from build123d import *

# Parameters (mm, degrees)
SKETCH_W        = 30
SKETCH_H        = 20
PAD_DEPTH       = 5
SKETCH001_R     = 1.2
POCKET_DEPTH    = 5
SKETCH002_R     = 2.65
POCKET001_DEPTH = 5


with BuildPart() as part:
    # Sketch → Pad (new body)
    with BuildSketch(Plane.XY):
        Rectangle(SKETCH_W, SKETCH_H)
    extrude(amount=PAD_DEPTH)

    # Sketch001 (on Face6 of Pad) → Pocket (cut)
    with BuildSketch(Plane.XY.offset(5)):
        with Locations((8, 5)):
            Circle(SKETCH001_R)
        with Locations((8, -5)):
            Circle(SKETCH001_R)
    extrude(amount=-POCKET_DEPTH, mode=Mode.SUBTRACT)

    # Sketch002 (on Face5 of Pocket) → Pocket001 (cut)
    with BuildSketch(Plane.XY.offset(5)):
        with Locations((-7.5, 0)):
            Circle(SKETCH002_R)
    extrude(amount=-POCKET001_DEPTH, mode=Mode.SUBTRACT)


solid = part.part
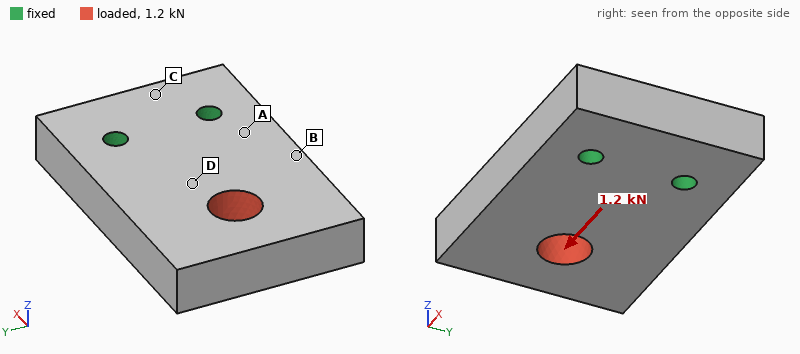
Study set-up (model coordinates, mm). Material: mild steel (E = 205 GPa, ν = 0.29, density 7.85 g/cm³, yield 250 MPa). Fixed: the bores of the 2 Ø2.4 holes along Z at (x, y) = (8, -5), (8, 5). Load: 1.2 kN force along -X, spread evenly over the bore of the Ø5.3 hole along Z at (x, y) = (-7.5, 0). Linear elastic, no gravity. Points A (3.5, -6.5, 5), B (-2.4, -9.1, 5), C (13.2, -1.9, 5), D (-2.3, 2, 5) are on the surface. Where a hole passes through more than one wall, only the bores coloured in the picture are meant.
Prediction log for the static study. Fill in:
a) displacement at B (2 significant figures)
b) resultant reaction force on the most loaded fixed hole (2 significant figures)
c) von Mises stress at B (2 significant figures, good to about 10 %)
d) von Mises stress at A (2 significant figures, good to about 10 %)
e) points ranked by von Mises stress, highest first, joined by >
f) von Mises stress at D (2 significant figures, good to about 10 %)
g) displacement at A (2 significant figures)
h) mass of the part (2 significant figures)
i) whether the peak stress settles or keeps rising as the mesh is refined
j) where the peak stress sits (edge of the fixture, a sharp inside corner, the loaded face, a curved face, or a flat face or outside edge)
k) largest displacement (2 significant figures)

0.69 µm
610 N
7.2 MPa
13 MPa
D > A > B > C
17 MPa
0.36 µm
22 g
keeps rising
edge of the fixture
1.7 µm
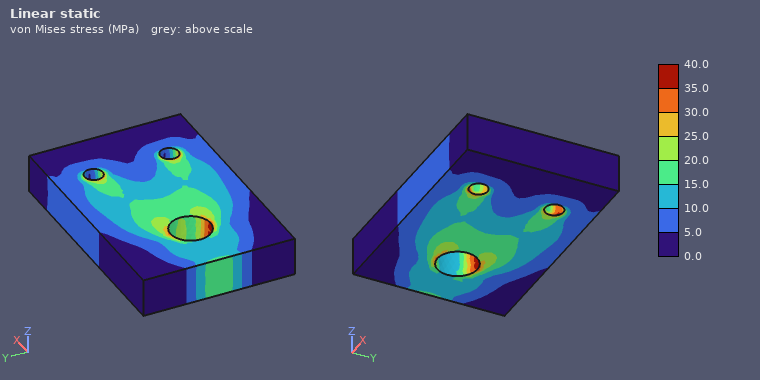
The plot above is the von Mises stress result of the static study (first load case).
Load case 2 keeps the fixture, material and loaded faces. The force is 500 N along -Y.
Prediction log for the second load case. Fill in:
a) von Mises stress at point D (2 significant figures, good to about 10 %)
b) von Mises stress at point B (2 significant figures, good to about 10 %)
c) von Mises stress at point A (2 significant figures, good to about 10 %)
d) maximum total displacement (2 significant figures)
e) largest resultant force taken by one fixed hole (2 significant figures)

14 MPa
7.8 MPa
13 MPa
4.1 µm
710 N
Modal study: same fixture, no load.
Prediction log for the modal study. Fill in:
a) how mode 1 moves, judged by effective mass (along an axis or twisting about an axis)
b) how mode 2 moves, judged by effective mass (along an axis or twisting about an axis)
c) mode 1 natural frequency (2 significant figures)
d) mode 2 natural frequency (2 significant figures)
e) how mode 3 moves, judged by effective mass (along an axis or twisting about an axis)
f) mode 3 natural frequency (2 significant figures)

along Z
twisting about X
7600 Hz
17 kHz
along Y
19 kHz
